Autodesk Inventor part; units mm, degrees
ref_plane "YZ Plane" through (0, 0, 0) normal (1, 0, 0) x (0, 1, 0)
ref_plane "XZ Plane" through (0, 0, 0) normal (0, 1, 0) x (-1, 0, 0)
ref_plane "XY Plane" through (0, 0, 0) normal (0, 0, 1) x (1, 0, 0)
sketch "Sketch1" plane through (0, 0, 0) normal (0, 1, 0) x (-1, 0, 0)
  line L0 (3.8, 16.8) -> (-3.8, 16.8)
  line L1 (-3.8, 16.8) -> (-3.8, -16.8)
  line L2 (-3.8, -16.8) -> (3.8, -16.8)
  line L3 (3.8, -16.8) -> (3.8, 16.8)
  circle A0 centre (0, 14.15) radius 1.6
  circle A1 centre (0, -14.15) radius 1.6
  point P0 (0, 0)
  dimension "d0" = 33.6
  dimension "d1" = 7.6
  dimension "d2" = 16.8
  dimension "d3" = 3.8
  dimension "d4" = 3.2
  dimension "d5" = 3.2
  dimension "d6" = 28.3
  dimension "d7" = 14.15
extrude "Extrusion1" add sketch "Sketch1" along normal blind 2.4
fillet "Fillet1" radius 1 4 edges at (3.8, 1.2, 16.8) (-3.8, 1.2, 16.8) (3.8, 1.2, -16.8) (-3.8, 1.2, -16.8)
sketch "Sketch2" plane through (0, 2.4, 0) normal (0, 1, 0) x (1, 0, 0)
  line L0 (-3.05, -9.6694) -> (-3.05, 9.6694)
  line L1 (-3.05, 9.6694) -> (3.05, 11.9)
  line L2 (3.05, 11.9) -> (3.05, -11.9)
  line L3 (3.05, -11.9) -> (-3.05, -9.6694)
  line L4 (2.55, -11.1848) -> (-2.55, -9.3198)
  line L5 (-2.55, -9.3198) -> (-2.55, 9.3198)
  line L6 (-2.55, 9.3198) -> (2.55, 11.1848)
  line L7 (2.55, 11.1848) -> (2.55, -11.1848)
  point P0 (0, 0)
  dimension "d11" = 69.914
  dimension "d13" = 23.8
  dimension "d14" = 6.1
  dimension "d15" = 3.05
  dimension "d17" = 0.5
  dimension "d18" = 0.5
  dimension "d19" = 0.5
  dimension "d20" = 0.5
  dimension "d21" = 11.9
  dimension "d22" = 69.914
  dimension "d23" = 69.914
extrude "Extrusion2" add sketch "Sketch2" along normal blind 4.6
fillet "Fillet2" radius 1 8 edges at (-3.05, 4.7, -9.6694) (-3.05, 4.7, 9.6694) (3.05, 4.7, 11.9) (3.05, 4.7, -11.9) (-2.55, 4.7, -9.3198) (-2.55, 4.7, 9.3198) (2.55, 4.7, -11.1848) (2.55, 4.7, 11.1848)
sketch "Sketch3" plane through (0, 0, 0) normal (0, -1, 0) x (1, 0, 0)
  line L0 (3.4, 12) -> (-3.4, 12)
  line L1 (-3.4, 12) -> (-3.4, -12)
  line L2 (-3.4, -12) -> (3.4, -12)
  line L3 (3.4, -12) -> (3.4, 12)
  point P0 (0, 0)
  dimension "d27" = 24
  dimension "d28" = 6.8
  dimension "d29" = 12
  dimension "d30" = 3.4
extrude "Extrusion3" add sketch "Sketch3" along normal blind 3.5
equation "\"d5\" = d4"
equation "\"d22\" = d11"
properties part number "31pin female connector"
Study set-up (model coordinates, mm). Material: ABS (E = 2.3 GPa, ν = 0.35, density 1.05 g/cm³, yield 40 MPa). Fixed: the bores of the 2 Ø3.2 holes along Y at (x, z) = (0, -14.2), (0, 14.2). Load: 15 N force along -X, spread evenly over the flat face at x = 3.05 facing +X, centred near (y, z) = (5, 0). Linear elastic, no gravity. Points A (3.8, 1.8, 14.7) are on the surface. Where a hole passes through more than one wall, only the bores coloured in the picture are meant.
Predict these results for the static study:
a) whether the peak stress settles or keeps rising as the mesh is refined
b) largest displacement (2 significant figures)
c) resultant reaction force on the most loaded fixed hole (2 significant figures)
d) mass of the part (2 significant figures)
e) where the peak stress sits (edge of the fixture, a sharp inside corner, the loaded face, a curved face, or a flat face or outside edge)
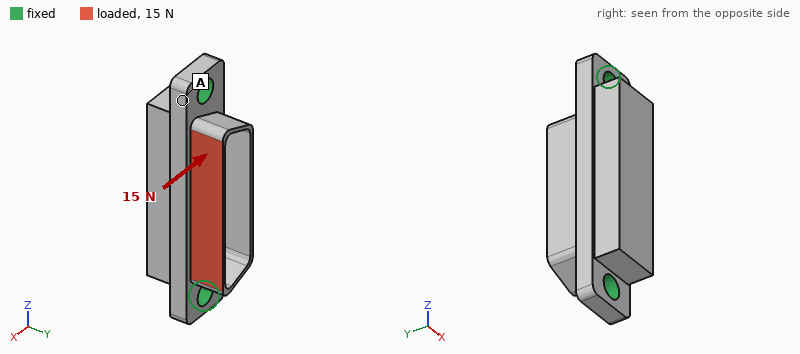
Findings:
keeps rising
0.34 mm
7.6 N
1.3 g
a sharp inside corner
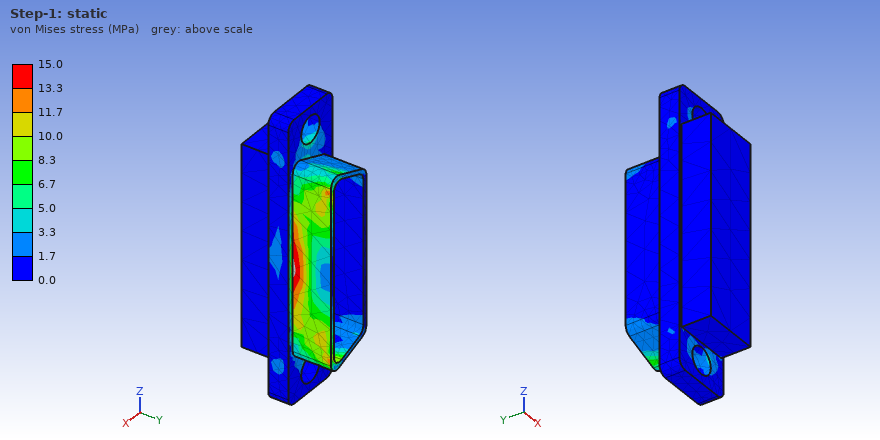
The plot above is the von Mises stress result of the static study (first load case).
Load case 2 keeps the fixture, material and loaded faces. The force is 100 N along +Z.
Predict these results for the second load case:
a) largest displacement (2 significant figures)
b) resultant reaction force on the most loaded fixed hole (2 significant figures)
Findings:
47 µm
53 N
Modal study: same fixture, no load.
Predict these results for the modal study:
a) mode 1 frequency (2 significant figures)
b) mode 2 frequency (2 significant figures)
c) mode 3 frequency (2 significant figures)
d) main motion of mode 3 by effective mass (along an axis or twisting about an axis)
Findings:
6000 Hz
6600 Hz
7000 Hz
along X
